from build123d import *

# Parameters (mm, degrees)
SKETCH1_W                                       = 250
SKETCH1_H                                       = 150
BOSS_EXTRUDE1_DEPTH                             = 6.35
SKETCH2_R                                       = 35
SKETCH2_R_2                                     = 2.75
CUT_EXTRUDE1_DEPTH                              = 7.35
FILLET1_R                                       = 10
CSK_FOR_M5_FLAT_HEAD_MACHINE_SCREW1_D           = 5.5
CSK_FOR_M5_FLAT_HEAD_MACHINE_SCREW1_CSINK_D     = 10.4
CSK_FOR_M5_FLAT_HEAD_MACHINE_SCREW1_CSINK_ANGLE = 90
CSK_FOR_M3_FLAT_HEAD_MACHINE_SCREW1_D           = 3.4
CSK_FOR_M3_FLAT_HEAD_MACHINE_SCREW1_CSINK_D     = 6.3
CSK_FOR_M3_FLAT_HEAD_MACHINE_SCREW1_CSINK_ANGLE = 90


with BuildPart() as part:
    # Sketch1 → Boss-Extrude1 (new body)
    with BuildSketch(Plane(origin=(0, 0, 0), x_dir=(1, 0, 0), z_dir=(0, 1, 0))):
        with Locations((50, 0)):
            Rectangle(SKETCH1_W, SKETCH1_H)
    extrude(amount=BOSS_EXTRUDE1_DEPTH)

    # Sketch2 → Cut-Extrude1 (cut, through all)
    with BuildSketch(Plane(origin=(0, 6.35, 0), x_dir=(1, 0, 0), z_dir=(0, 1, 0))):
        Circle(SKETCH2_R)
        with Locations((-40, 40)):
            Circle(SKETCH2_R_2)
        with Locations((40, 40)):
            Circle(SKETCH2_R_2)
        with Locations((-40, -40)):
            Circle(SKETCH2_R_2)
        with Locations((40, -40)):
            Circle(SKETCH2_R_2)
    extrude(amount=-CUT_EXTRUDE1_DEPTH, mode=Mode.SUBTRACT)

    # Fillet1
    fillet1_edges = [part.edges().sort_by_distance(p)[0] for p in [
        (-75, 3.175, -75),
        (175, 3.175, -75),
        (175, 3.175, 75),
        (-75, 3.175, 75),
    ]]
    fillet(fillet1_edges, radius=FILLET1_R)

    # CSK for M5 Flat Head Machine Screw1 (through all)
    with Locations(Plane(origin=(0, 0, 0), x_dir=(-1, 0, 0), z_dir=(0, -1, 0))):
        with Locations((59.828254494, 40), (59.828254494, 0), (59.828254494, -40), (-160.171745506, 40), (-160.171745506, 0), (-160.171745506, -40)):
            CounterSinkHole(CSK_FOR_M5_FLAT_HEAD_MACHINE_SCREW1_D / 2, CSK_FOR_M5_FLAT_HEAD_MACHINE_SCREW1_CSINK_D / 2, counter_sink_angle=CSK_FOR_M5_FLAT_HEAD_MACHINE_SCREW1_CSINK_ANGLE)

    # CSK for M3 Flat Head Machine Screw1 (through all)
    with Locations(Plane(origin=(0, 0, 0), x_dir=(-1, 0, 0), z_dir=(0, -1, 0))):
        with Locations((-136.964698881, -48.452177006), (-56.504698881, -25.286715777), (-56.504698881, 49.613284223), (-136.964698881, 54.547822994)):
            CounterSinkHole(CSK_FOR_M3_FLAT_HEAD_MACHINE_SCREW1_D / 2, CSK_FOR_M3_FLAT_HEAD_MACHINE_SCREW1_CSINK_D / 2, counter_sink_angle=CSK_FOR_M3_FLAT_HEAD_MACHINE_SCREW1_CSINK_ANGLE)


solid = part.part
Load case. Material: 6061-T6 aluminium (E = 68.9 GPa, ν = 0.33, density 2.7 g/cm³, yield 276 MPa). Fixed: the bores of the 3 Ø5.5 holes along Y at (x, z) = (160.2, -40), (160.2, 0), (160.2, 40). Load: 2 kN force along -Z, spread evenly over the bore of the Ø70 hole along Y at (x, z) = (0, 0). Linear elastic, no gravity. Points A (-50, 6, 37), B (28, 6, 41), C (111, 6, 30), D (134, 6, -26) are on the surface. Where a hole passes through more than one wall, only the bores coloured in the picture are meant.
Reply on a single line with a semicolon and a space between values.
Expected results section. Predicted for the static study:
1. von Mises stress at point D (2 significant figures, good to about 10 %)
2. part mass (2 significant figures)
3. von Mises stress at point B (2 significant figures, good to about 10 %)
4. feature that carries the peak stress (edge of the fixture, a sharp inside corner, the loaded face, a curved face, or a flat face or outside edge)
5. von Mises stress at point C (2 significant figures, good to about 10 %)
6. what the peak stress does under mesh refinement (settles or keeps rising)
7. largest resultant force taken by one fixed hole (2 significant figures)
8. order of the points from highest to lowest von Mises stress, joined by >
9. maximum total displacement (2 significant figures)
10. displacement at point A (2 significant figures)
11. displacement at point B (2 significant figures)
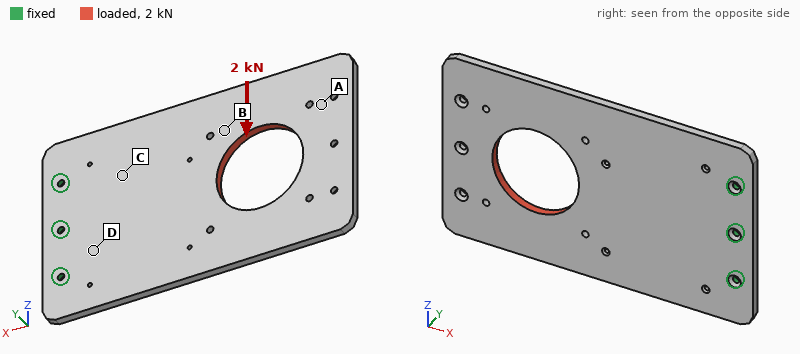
13 MPa; 570 g; 4.8 MPa; edge of the fixture; 8.4 MPa; keeps rising; 3.9 kN; D > C > B > A; 0.12 mm; 0.11 mm; 0.064 mm
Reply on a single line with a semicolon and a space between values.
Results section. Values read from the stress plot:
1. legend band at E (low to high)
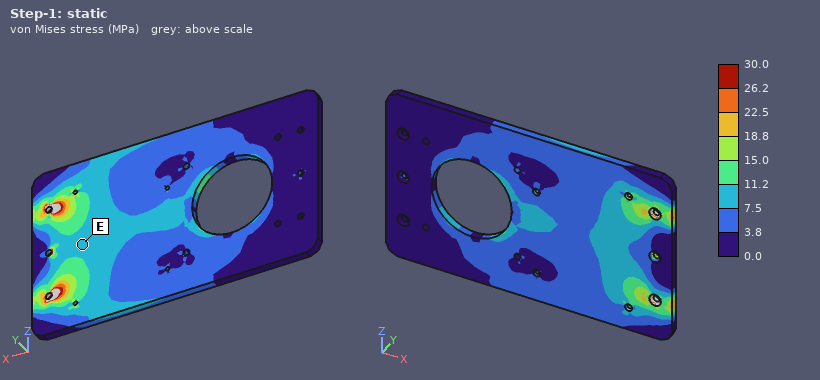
7.5 to 11.2 MPa
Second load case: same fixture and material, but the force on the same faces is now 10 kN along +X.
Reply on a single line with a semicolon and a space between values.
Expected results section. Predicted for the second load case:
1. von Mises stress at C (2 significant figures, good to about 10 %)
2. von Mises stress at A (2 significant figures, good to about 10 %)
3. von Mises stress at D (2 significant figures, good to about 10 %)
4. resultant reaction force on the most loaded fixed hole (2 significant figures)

12 MPa; 7.4 MPa; 12 MPa; 3.6 kN
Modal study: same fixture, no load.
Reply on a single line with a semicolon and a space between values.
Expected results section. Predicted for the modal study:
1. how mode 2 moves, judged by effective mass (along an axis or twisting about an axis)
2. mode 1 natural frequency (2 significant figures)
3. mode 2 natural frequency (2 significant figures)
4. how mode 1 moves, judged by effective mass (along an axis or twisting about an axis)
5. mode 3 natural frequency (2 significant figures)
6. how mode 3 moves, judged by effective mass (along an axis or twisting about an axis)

twisting about X; 94 Hz; 290 Hz; along Y; 510 Hz; along Y
